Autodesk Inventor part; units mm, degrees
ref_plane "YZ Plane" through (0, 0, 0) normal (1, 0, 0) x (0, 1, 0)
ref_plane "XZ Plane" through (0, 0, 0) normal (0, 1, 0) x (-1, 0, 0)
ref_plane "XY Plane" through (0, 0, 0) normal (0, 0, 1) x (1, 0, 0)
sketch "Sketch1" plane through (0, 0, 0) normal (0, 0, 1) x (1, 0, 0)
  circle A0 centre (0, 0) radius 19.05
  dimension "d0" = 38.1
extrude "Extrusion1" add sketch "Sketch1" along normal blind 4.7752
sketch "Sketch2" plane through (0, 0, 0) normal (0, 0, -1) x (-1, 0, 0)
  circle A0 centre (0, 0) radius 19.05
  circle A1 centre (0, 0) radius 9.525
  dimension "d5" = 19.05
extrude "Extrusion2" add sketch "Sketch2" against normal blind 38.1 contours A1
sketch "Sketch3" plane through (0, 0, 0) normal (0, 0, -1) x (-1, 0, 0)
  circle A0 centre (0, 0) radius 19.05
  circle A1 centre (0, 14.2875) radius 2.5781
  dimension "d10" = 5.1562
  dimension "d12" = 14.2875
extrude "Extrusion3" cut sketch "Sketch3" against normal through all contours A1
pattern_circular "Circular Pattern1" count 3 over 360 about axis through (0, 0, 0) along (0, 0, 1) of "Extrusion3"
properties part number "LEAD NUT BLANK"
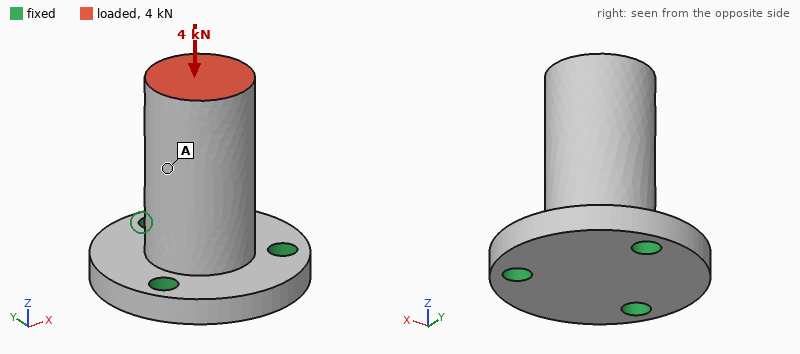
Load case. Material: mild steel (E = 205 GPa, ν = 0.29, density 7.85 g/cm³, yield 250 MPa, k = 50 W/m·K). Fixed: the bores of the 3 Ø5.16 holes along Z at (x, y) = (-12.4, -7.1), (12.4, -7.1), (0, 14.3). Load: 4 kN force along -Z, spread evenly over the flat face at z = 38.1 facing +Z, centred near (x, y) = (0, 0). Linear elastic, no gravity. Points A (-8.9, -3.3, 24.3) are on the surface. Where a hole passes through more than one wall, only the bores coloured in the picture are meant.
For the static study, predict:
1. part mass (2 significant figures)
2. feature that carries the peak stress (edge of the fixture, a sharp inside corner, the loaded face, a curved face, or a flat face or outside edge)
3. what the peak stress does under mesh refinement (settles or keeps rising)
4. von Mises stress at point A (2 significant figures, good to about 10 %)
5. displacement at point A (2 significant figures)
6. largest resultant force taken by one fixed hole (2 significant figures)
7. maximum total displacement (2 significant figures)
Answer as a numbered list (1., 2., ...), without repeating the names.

1. 110 g
2. edge of the fixture
3. keeps rising
4. 14 MPa
5. 3.9 µm
6. 1.4 kN
7. 4.8 µm
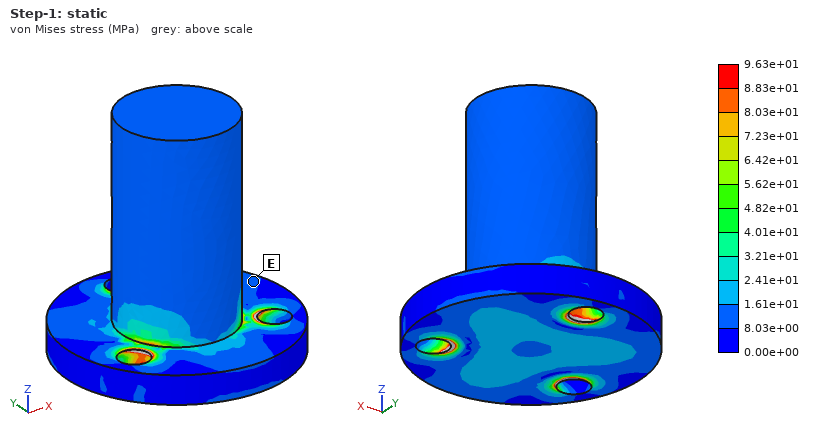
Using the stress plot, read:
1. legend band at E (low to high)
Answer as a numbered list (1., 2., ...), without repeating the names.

1. 8.03e+00 to 1.61e+01 MPa
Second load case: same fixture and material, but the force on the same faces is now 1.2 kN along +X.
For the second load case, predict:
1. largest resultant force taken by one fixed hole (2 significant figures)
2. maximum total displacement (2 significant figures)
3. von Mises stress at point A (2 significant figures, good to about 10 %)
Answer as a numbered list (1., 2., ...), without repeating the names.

1. 1.9 kN
2. 29 µm
3. 23 MPa
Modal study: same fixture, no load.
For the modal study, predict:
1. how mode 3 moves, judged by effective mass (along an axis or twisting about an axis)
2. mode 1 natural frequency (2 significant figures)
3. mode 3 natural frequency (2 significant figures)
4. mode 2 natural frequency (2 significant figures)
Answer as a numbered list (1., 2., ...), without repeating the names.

1. along Z
2. 6800 Hz
3. 19 kHz
4. 6800 Hz
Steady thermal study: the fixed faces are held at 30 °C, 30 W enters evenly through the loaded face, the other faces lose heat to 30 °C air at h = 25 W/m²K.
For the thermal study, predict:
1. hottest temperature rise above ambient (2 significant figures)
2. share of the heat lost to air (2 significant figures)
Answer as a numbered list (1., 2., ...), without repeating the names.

1. 84 K
2. 9.6 %
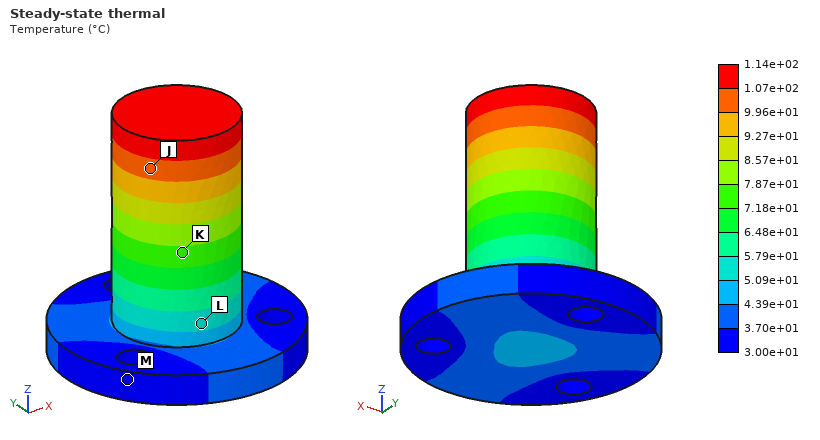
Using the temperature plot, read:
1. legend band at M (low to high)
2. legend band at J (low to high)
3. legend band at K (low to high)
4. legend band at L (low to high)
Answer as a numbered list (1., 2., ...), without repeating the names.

1. 3.00e+01 to 3.70e+01 °C
2. 9.96e+01 to 1.07e+02 °C
3. 7.18e+01 to 7.87e+01 °C
4. 5.09e+01 to 5.79e+01 °C
